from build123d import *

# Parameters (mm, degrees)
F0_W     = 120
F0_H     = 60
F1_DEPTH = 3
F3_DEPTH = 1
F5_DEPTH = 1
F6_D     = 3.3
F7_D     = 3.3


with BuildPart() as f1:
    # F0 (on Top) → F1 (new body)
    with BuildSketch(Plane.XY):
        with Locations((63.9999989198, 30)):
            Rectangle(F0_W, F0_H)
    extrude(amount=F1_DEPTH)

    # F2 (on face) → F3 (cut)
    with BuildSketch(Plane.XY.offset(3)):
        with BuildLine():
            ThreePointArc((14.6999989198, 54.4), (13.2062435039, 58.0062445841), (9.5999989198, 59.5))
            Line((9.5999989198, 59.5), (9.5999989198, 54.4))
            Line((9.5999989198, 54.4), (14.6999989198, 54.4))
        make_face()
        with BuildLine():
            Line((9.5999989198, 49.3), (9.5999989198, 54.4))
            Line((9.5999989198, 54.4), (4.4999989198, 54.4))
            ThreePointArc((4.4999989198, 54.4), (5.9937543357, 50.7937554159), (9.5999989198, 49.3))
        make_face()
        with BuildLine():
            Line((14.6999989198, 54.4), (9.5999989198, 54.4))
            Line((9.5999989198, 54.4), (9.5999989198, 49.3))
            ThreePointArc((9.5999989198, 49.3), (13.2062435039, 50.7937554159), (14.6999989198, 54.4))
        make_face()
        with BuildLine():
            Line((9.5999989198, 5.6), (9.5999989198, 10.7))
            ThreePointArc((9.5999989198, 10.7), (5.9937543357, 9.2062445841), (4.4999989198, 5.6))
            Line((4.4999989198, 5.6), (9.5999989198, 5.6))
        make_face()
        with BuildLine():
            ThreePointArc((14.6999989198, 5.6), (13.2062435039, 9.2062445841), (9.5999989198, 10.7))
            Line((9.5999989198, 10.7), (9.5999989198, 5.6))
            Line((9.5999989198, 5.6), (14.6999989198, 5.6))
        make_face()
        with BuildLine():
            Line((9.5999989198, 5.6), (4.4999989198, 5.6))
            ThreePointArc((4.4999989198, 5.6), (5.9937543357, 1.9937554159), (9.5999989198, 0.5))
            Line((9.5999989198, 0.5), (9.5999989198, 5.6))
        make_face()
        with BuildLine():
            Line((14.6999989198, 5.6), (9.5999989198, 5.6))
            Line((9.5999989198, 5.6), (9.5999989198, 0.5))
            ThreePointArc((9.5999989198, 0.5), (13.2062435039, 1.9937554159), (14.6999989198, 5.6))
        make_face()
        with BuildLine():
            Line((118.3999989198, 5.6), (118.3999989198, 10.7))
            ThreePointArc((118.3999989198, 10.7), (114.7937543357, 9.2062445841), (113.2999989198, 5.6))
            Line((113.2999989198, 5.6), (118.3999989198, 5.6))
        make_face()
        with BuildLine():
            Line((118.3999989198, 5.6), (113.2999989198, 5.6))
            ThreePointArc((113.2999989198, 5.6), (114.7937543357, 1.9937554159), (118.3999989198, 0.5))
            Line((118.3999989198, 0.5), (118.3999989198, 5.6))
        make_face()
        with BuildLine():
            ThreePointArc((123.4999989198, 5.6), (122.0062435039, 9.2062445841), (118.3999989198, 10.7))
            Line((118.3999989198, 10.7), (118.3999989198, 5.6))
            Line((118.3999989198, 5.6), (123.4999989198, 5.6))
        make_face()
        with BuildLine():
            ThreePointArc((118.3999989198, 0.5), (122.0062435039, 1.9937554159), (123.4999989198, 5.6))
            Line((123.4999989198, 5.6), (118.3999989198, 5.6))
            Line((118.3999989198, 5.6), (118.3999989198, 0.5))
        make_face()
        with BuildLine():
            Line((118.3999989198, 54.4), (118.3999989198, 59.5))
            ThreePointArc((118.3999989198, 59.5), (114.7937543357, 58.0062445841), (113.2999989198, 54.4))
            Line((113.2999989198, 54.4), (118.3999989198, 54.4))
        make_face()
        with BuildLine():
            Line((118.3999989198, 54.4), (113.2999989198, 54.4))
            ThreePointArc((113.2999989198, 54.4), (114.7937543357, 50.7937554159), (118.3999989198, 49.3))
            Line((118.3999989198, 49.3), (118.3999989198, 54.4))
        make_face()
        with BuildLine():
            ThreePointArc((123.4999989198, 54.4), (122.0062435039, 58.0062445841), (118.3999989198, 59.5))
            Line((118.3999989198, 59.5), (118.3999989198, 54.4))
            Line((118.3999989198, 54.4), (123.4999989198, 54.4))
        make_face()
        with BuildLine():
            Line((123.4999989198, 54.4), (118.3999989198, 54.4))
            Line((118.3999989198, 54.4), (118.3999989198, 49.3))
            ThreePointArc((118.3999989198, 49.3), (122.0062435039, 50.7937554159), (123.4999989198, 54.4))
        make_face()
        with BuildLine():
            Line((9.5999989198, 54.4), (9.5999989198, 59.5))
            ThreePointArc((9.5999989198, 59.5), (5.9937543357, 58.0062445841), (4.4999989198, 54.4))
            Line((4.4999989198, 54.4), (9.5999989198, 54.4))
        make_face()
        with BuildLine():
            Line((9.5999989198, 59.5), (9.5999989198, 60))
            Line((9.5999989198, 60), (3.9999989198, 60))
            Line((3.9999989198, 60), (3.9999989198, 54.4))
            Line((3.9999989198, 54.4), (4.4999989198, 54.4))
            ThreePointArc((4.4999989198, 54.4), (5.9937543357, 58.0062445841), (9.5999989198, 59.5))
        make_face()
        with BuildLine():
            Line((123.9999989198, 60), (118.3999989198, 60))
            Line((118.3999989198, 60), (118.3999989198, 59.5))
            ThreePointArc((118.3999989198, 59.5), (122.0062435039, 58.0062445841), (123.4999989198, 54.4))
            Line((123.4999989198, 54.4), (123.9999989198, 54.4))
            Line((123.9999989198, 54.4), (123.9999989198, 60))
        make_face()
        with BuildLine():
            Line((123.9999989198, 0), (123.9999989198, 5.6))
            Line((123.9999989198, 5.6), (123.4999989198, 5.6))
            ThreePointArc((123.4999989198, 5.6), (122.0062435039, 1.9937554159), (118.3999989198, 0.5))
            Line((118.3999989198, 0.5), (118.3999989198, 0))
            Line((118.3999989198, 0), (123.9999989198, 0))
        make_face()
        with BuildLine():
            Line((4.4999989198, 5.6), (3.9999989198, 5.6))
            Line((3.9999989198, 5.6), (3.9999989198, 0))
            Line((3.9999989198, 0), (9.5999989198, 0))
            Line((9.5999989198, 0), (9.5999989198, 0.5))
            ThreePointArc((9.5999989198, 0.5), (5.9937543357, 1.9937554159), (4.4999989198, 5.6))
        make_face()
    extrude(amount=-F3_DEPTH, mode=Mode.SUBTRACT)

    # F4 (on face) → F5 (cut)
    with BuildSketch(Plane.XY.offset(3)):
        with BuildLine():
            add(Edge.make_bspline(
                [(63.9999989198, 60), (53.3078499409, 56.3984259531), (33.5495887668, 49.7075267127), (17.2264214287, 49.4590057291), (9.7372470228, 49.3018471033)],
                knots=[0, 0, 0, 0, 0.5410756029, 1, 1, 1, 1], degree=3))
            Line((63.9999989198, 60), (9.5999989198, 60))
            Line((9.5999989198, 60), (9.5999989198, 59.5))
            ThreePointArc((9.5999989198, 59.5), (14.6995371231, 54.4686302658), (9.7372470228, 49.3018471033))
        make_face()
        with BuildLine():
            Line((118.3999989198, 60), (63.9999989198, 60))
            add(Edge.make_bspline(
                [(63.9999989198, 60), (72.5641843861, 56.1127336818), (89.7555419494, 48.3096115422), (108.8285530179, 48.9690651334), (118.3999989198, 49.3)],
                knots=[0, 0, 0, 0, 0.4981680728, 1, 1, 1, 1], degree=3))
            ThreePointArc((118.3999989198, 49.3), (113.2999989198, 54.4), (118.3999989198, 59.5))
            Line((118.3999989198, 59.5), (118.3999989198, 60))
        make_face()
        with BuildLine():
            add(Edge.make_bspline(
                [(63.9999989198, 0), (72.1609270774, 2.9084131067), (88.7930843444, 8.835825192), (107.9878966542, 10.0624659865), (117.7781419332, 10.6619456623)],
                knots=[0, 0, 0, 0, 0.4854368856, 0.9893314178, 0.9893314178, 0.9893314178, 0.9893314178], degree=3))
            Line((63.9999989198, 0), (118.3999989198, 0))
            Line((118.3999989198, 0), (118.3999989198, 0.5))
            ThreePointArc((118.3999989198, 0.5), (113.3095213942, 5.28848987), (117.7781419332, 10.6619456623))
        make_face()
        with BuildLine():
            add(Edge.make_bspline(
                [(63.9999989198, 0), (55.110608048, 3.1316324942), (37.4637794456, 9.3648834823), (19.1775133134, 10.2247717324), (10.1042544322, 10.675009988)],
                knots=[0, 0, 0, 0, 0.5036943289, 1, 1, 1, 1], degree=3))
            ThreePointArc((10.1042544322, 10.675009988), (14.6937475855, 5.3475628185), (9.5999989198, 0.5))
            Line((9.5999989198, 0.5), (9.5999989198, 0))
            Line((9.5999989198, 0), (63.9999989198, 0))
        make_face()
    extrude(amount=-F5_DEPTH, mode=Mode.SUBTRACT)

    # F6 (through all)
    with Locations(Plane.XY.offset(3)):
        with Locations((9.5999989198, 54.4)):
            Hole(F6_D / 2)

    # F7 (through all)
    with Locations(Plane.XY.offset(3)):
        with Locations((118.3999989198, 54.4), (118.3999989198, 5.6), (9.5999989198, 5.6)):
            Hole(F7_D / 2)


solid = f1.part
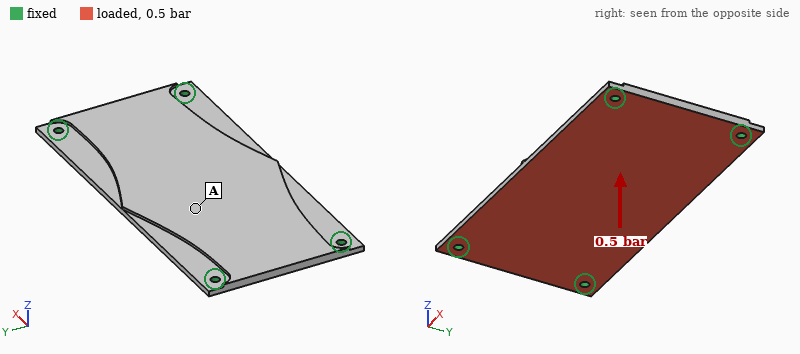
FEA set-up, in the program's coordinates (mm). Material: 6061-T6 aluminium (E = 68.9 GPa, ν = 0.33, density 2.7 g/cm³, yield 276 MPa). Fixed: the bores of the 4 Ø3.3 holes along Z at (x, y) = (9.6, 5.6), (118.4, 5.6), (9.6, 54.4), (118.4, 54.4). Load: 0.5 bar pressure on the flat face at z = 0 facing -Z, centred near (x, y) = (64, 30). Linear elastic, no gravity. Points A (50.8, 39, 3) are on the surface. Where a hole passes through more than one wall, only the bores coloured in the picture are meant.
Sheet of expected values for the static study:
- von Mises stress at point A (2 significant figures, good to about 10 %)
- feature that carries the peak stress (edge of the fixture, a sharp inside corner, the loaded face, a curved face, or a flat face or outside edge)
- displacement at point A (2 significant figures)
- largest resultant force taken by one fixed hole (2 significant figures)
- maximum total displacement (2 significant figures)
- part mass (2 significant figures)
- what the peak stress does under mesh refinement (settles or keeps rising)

22 MPa
edge of the fixture
0.21 mm
190 N
0.24 mm
53 g
keeps rising
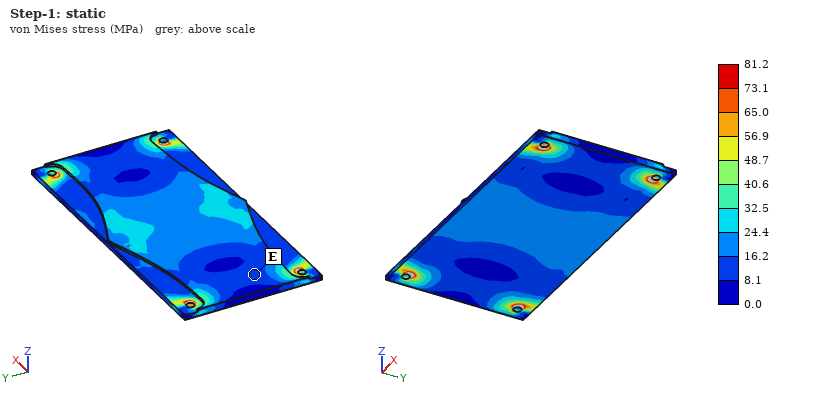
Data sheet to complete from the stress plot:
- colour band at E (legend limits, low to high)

8.1 to 16.2 MPa
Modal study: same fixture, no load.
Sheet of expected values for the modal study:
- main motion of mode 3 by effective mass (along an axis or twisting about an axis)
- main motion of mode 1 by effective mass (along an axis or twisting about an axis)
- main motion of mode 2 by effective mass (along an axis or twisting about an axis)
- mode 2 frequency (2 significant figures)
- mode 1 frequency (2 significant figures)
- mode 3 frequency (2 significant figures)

twisting about Y
along Z
twisting about X
1800 Hz
960 Hz
2800 Hz
